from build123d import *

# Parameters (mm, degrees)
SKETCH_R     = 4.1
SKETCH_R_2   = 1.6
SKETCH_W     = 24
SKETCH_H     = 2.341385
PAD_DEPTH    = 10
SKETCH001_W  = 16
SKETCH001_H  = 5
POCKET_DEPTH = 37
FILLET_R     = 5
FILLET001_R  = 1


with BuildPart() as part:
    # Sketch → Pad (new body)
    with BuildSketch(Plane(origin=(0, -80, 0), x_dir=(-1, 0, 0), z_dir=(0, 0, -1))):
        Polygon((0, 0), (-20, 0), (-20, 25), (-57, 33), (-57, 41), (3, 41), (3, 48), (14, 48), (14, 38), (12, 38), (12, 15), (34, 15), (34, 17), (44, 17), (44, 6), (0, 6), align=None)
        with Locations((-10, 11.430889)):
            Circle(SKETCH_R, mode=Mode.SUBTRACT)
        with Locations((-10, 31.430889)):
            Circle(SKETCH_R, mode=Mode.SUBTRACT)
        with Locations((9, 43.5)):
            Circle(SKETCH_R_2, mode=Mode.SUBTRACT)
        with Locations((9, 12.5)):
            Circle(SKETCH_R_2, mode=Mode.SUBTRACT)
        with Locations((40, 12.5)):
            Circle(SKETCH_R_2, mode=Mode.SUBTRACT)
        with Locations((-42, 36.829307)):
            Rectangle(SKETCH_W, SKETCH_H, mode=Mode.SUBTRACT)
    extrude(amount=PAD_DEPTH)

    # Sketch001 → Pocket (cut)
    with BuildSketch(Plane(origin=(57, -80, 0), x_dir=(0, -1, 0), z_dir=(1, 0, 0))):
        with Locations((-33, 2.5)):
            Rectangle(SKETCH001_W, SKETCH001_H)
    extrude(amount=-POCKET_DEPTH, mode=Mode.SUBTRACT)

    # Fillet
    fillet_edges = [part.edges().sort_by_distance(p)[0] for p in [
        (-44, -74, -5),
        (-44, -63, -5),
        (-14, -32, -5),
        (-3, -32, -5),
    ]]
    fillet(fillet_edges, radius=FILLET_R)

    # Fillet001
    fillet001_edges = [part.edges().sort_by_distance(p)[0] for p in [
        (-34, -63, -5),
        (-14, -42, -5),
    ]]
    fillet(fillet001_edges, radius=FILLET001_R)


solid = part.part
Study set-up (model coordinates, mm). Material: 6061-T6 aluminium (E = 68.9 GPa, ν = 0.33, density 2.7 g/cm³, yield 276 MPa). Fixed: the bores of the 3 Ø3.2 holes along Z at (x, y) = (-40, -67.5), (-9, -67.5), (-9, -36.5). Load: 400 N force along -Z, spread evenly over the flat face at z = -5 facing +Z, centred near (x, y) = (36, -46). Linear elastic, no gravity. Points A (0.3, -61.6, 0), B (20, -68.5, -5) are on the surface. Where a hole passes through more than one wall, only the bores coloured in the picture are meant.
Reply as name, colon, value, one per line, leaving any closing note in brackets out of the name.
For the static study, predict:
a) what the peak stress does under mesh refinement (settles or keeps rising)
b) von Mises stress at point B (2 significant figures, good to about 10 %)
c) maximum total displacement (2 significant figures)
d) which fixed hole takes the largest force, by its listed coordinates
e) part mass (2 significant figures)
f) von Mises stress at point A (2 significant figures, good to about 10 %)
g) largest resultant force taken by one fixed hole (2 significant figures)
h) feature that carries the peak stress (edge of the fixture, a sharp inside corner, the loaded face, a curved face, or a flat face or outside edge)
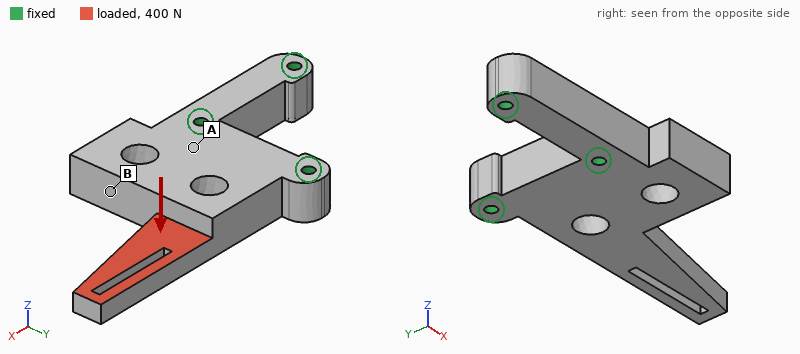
what the peak stress does under mesh refinement: keeps rising
von Mises stress at point B: 12 MPa
maximum total displacement: 0.46 mm
which fixed hole takes the largest force, by its listed coordinates: (-9, -36.5)
part mass: 45 g
von Mises stress at point A: 28 MPa
largest resultant force taken by one fixed hole: 280 N
feature that carries the peak stress: edge of the fixture
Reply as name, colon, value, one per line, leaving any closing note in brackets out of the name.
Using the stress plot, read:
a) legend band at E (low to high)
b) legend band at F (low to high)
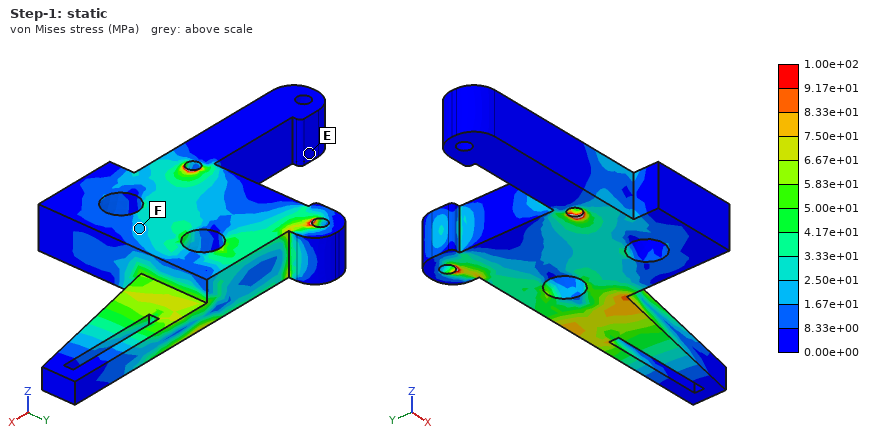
legend band at E: 0.00e+00 to 8.33e+00 MPa
legend band at F: 1.67e+01 to 2.50e+01 MPa
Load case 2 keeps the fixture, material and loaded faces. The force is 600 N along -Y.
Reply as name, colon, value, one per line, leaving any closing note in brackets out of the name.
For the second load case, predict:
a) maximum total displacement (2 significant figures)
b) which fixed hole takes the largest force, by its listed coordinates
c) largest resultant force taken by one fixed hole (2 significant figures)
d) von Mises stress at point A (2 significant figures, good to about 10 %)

maximum total displacement: 0.13 mm
which fixed hole takes the largest force, by its listed coordinates: (-9, -36.5)
largest resultant force taken by one fixed hole: 930 N
von Mises stress at point A: 7.6 MPa
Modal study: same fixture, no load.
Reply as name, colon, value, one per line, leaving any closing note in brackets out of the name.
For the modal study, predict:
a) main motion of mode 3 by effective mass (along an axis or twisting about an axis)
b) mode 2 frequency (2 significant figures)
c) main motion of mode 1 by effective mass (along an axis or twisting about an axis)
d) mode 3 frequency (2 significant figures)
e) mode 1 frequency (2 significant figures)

main motion of mode 3 by effective mass: along Z
mode 2 frequency: 6200 Hz
main motion of mode 1 by effective mass: along Z
mode 3 frequency: 6700 Hz
mode 1 frequency: 2600 Hz
